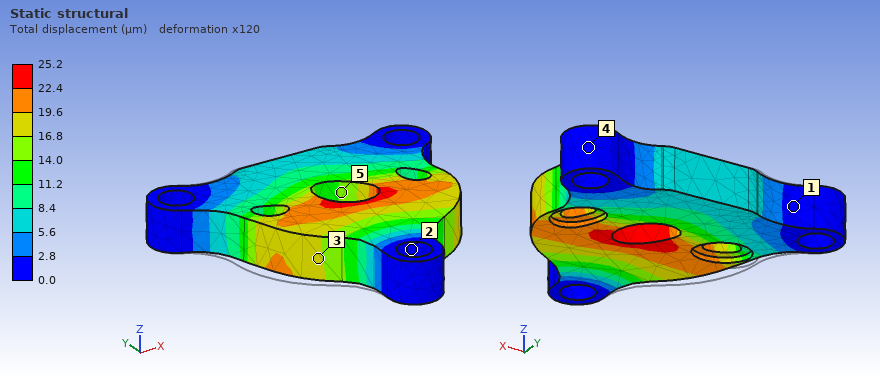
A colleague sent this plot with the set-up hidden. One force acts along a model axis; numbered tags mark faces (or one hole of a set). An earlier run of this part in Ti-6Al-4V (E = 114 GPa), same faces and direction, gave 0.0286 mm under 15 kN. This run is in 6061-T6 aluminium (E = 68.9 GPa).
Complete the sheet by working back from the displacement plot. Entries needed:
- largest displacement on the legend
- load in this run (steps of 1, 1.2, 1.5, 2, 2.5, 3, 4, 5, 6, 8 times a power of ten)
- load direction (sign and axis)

25.2 µm
8 kN
+X
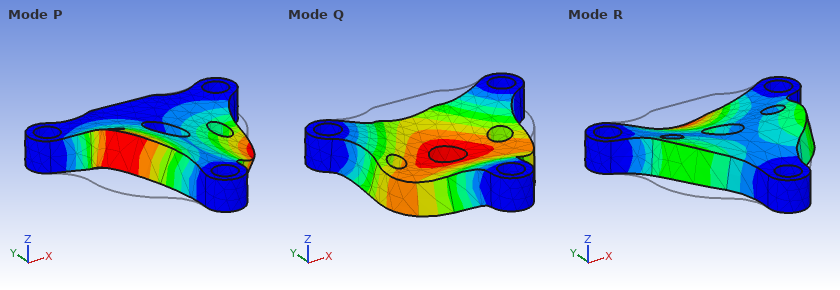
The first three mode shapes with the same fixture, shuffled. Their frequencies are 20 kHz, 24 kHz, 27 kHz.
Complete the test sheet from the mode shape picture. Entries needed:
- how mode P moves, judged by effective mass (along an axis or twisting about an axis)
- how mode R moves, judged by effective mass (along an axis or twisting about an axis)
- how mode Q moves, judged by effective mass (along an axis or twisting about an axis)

twisting about Y
twisting about X
along Z
